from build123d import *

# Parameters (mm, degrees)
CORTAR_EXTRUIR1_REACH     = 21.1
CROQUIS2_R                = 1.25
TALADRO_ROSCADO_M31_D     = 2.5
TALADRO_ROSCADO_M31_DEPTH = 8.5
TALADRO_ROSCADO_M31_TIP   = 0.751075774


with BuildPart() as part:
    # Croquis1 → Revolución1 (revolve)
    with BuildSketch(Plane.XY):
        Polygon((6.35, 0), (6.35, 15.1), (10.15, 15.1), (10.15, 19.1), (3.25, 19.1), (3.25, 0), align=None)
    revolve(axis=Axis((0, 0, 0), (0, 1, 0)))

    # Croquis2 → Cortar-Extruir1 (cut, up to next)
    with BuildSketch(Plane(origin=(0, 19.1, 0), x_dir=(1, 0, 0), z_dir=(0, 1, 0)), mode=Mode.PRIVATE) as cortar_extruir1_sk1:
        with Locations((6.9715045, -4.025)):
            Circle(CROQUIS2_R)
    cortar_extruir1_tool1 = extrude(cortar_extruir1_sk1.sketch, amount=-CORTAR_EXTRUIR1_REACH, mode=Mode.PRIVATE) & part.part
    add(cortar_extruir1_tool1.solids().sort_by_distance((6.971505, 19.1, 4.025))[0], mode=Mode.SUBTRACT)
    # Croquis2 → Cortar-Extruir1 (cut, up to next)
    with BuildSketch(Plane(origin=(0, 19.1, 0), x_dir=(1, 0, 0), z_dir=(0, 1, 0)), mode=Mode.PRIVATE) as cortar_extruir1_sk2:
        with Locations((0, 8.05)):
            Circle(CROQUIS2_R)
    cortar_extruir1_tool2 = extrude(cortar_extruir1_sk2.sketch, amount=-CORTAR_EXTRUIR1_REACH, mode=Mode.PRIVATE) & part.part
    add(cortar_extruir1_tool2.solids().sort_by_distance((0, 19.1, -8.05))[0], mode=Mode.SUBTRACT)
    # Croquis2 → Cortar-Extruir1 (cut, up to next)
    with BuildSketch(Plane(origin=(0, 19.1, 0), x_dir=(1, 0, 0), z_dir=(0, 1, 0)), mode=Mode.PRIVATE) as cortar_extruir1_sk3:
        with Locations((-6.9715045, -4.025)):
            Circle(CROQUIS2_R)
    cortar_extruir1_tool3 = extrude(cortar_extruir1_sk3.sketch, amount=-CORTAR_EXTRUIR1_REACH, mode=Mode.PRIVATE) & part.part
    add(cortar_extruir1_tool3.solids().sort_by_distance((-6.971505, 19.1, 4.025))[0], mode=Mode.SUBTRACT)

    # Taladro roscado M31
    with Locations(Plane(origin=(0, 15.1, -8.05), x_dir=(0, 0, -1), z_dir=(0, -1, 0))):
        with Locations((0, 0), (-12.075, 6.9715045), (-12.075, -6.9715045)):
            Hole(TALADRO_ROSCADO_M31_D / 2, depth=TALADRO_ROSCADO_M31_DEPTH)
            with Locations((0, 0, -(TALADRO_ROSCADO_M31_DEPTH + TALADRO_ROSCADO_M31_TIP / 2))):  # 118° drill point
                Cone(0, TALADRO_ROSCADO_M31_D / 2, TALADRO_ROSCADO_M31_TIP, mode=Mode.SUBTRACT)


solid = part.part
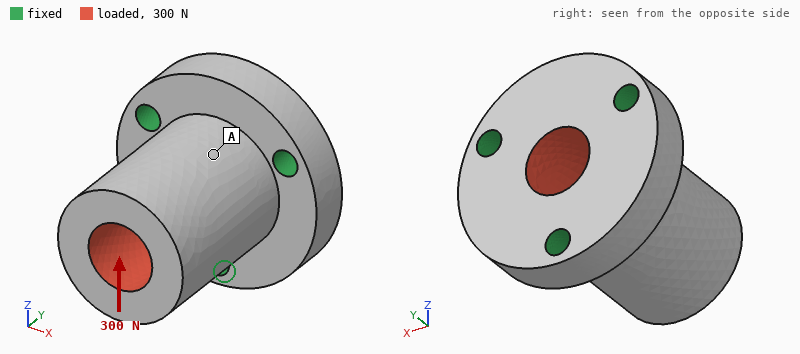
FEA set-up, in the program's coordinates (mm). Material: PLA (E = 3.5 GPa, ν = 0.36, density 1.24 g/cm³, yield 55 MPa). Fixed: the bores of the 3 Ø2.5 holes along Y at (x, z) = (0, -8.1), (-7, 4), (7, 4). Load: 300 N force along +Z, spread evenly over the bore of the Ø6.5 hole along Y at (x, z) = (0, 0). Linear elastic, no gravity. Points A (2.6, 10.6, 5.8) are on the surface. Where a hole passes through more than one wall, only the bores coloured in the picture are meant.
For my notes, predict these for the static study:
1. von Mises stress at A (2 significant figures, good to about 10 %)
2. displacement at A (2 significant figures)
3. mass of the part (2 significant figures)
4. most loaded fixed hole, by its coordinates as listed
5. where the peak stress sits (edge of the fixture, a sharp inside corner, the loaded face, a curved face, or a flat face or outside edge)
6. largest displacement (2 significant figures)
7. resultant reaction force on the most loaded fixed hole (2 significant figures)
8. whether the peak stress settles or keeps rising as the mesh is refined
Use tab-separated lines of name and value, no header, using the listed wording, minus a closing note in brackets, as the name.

von Mises stress at A	3.6 MPa
displacement at A	44 µm
mass of the part	3.1 g
most loaded fixed hole, by its coordinates as listed	(0, -8.1)
where the peak stress sits	a sharp inside corner
largest displacement	99 µm
resultant reaction force on the most loaded fixed hole	210 N
whether the peak stress settles or keeps rising as the mesh is refined	keeps rising
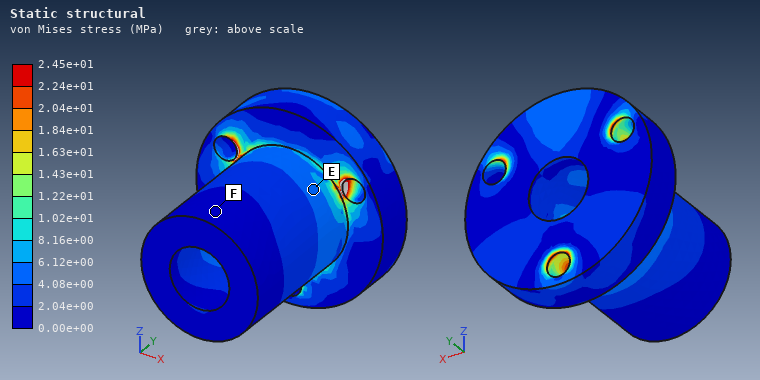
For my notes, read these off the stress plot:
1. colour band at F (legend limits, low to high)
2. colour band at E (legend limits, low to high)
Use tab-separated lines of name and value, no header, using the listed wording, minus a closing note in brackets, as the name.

colour band at F	0.00e+00 to 2.04e+00 MPa
colour band at E	4.08e+00 to 6.12e+00 MPa
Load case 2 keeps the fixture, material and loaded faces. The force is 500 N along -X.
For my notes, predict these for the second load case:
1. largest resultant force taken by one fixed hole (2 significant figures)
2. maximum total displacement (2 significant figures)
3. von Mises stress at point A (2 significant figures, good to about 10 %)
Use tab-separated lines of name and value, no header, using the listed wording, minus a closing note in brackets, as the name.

largest resultant force taken by one fixed hole	310 N
maximum total displacement	0.17 mm
von Mises stress at point A	7.9 MPa
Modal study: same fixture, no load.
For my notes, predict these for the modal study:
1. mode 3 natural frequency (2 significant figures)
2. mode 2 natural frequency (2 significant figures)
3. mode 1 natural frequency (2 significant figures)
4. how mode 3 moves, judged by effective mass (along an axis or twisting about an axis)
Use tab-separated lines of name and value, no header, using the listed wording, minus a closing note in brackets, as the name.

mode 3 natural frequency	15 kHz
mode 2 natural frequency	6900 Hz
mode 1 natural frequency	6900 Hz
how mode 3 moves, judged by effective mass	twisting about Y
